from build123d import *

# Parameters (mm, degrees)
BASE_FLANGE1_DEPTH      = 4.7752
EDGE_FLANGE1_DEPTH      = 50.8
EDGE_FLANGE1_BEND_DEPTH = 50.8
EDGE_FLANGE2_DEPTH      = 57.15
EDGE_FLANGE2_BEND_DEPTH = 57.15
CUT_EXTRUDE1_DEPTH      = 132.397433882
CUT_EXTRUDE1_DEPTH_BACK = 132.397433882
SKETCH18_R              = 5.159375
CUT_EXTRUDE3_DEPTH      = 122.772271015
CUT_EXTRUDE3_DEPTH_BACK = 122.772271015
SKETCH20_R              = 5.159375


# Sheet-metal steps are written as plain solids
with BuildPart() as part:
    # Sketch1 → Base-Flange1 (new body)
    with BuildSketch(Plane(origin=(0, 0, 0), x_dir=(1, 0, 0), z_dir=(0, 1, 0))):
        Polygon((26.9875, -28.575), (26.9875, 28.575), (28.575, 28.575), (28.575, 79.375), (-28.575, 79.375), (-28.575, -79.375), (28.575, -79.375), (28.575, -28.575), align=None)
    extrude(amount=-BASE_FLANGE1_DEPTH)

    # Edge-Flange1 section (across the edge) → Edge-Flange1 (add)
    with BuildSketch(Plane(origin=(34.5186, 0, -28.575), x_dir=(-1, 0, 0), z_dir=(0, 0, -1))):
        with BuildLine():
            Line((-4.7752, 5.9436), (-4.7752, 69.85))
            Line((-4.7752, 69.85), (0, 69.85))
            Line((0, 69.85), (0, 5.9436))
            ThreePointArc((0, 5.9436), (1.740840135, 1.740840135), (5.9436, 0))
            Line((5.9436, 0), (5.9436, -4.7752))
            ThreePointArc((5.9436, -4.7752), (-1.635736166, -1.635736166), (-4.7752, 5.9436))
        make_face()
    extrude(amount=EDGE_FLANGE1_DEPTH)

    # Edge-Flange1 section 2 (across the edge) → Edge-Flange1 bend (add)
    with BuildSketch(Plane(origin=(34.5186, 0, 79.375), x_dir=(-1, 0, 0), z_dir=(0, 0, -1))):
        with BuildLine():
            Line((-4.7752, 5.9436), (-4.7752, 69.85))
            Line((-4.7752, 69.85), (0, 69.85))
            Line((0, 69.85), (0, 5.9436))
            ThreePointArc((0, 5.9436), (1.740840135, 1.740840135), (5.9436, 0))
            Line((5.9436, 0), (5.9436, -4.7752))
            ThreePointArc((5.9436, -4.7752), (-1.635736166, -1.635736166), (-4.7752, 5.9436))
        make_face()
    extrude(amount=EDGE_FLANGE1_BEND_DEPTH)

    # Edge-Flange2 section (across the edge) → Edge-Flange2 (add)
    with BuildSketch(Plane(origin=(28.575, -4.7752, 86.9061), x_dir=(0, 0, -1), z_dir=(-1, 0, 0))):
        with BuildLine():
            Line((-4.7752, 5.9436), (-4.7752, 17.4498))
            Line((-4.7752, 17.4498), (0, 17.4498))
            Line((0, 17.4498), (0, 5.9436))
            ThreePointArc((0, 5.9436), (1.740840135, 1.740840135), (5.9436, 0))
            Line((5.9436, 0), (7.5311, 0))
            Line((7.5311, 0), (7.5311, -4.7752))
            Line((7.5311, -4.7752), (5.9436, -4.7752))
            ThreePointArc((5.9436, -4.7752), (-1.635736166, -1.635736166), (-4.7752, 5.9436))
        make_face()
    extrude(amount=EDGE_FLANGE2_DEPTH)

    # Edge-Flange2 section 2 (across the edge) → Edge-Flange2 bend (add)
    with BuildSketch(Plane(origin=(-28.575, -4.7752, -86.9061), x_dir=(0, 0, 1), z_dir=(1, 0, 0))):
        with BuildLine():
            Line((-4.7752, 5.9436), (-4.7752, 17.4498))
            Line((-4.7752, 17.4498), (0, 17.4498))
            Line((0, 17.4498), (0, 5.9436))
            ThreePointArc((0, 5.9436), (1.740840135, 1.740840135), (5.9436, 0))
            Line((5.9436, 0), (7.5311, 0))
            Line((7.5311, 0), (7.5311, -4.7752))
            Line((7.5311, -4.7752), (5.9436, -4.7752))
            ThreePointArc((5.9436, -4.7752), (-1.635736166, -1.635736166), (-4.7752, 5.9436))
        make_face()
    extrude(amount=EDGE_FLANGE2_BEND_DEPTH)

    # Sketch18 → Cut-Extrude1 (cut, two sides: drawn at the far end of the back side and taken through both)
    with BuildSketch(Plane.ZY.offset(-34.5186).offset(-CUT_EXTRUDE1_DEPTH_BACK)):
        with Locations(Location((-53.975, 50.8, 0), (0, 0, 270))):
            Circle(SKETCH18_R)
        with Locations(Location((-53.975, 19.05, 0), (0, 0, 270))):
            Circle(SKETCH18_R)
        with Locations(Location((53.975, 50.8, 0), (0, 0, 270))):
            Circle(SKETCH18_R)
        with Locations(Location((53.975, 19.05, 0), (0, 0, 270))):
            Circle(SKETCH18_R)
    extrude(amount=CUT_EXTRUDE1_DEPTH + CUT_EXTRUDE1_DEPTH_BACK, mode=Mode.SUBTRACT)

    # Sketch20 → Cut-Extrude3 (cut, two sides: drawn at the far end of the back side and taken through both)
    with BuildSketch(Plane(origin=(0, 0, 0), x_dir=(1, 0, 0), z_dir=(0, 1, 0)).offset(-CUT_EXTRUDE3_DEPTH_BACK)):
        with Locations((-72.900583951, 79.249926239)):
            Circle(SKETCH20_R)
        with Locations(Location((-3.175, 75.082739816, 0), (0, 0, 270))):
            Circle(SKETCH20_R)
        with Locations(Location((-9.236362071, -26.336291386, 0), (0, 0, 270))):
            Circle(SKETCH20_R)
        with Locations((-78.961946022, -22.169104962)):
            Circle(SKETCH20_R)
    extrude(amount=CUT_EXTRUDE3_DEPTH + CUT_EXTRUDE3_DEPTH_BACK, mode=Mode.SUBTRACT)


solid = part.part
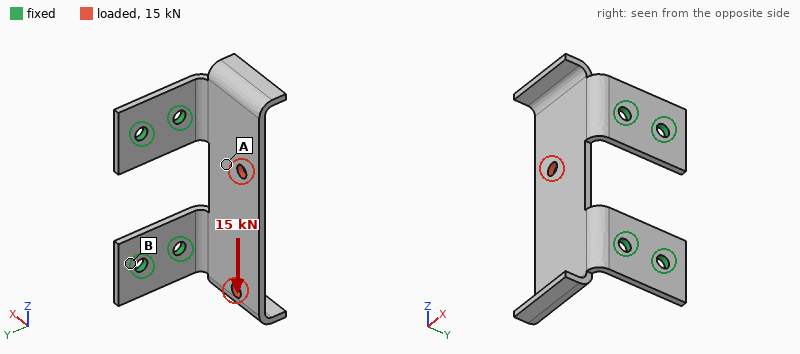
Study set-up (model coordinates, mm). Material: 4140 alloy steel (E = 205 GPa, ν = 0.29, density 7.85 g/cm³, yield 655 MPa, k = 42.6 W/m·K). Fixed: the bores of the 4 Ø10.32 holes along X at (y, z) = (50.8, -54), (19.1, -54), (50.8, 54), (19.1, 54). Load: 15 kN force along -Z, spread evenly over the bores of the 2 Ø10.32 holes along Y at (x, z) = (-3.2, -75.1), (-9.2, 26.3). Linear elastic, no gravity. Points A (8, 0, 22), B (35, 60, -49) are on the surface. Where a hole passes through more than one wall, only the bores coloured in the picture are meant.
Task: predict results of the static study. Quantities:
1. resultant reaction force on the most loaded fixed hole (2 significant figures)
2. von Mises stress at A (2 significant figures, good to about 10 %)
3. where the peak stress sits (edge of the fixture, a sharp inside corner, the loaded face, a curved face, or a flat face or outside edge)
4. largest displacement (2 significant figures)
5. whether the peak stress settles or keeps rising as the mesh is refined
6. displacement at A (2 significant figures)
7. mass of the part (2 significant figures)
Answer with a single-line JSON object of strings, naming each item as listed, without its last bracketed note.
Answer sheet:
{"resultant reaction force on the most loaded fixed hole": "12 kN", "von Mises stress at A": "120 MPa", "where the peak stress sits": "edge of the fixture", "largest displacement": "0.59 mm", "whether the peak stress settles or keeps rising as the mesh is refined": "keeps rising", "displacement at A": "0.14 mm", "mass of the part": "720 g"}
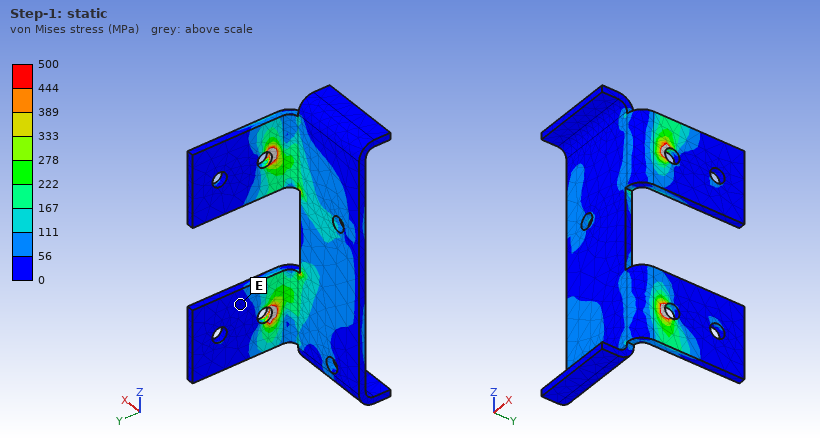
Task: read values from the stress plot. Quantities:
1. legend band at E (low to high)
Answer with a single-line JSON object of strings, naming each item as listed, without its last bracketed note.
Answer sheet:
{"legend band at E": "0 to 56 MPa"}
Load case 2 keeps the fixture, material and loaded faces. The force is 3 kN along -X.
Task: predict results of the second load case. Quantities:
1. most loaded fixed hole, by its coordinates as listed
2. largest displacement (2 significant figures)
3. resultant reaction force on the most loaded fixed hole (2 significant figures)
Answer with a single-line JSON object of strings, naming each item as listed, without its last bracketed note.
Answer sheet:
{"most loaded fixed hole, by its coordinates as listed": "(19.1, -54)", "largest displacement": "0.30 mm", "resultant reaction force on the most loaded fixed hole": "2.4 kN"}
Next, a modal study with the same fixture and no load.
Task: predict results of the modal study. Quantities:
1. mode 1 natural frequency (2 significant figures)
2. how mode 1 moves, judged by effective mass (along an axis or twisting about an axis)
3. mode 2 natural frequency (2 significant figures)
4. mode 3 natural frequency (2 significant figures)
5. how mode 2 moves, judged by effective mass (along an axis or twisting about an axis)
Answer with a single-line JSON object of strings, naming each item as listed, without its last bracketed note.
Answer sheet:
{"mode 1 natural frequency": "470 Hz", "how mode 1 moves, judged by effective mass": "along Y", "mode 2 natural frequency": "690 Hz", "mode 3 natural frequency": "1300 Hz", "how mode 2 moves, judged by effective mass": "twisting about X"}
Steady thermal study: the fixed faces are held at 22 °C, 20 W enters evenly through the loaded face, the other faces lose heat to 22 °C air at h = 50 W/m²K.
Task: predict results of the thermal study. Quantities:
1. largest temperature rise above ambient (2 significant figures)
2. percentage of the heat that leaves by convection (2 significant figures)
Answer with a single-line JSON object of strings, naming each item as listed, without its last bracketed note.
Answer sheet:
{"largest temperature rise above ambient": "27 K", "percentage of the heat that leaves by convection": "80 %"}
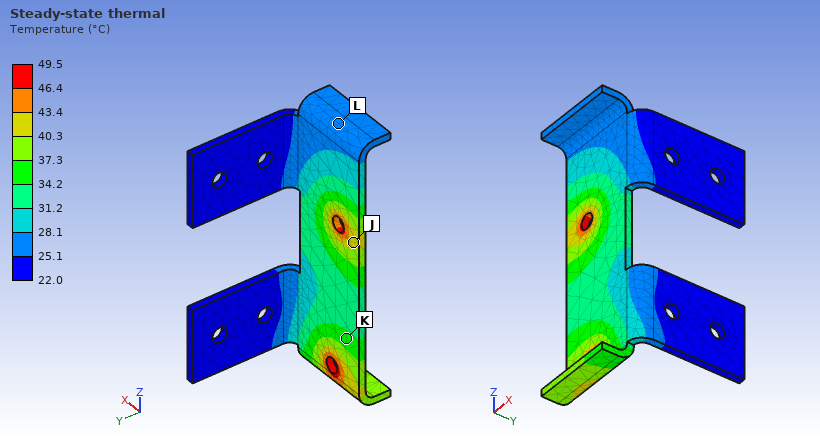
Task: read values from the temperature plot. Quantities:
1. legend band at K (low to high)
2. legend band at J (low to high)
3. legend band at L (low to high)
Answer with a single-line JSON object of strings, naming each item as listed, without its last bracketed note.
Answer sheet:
{"legend band at K": "34.2 to 37.3 °C", "legend band at J": "40.3 to 43.4 °C", "legend band at L": "25.1 to 28.1 °C"}
